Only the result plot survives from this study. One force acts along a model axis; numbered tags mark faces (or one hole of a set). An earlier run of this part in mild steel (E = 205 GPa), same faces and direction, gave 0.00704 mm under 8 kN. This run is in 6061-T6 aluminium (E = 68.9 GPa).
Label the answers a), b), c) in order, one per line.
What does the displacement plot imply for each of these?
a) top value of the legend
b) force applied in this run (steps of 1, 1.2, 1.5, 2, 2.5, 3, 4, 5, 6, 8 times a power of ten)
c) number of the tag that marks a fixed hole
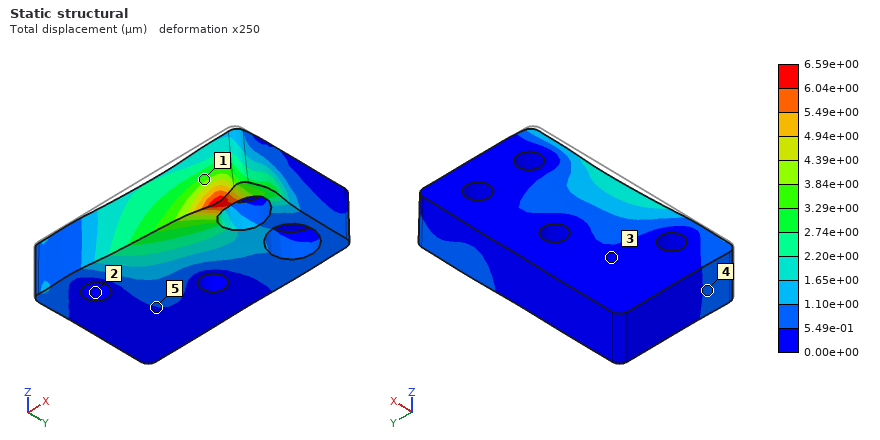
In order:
a) 6.59e+00 µm
b) 2.5 kN
c) 2
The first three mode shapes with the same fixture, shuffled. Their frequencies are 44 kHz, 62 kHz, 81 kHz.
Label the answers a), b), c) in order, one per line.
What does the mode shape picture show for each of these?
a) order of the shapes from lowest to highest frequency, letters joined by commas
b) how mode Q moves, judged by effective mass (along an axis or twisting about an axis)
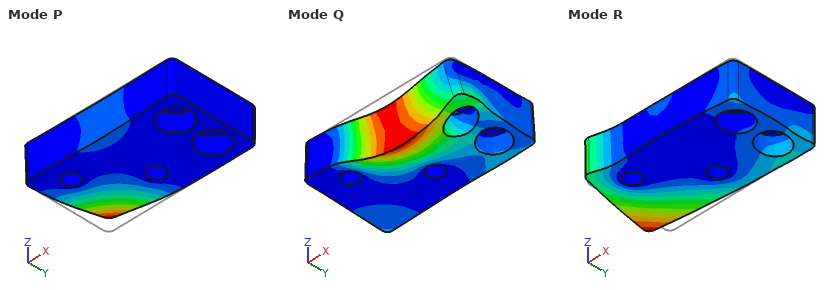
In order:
a) P, Q, R
b) along Z
